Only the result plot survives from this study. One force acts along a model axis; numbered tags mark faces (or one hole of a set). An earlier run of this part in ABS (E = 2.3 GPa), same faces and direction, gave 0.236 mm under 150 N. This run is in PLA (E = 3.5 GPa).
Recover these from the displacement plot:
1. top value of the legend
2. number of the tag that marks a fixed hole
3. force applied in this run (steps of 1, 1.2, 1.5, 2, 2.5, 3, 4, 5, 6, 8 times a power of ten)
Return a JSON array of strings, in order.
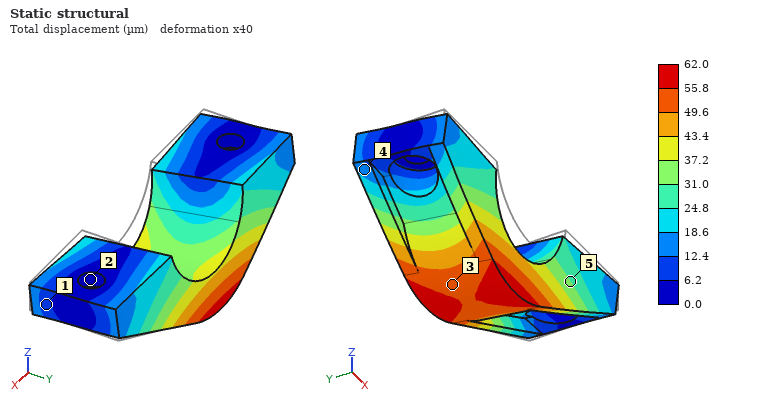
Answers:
["62.0 µm", "2", "60 N"]
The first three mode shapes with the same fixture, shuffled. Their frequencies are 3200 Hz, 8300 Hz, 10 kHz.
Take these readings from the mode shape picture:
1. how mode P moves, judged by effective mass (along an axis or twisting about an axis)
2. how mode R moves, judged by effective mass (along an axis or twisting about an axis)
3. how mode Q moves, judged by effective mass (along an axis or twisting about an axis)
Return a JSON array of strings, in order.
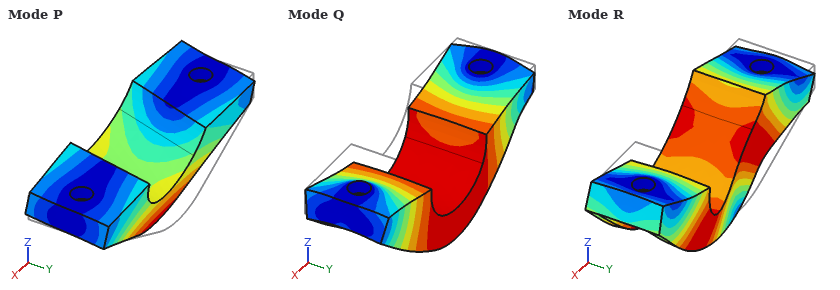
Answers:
["along Y", "along X", "along Z"]
